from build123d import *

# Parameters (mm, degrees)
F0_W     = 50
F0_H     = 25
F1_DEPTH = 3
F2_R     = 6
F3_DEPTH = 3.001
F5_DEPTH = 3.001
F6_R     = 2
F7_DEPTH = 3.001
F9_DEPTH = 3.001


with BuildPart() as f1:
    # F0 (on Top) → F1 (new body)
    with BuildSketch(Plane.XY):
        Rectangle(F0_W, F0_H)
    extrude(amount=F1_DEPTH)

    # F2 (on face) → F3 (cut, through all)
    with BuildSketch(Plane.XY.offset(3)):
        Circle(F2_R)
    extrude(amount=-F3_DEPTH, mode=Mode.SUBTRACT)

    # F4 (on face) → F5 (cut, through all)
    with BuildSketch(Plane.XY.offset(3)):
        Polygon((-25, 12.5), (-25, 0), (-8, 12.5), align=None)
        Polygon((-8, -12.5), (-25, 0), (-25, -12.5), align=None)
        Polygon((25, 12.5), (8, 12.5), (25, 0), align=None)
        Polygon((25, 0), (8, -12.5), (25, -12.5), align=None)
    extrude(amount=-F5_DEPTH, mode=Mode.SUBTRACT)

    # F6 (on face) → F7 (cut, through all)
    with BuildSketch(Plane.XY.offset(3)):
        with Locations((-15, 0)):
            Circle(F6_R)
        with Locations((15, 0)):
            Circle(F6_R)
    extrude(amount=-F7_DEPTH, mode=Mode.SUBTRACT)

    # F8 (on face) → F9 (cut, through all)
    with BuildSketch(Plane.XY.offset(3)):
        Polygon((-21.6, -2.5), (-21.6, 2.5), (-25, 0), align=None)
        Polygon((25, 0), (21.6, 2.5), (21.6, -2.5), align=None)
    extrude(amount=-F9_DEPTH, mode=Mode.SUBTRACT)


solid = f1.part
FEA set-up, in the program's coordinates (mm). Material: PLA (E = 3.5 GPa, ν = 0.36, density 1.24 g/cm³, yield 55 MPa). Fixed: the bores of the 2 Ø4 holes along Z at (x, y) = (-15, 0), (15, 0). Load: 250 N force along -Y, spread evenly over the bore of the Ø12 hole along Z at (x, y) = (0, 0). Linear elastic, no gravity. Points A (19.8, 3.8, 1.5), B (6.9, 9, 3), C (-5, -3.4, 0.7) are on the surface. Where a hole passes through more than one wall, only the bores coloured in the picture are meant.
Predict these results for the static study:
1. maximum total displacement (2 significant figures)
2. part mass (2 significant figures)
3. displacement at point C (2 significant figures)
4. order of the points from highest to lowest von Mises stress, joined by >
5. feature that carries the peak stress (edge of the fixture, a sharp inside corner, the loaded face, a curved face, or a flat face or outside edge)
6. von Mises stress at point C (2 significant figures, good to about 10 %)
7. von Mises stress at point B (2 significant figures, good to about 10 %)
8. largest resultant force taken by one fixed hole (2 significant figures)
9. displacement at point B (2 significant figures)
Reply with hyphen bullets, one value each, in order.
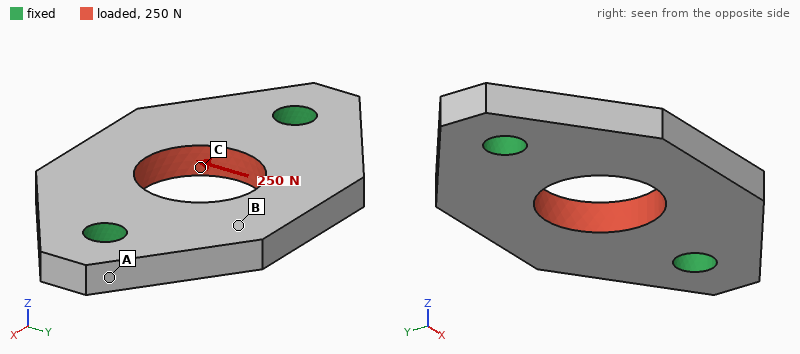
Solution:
- 28 µm
- 2.5 g
- 23 µm
- C > B > A
- edge of the fixture
- 4.6 MPa
- 3.2 MPa
- 130 N
- 19 µm
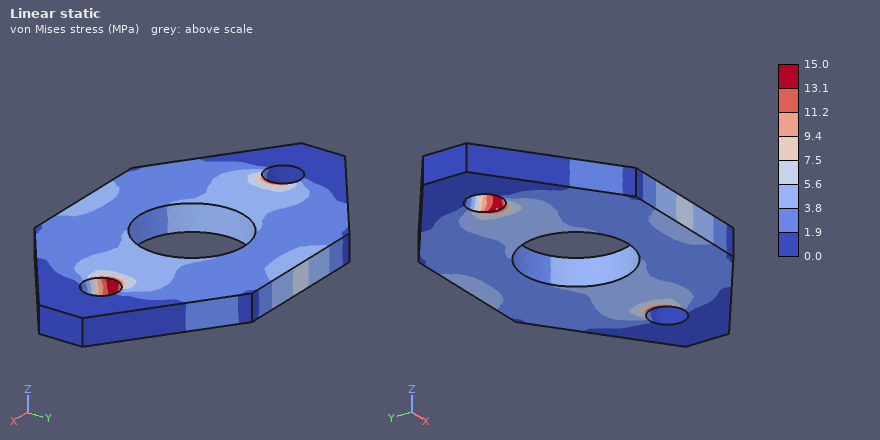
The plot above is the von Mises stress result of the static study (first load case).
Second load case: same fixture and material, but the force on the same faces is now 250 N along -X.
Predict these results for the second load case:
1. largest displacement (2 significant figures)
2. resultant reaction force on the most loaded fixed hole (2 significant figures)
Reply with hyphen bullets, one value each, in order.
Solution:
- 14 µm
- 130 N
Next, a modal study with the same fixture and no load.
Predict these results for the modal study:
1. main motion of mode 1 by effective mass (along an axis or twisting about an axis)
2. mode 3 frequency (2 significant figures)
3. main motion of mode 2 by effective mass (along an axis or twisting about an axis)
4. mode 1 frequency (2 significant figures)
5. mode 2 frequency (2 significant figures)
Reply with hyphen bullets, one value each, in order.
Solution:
- twisting about X
- 9000 Hz
- along Z
- 3800 Hz
- 4300 Hz
